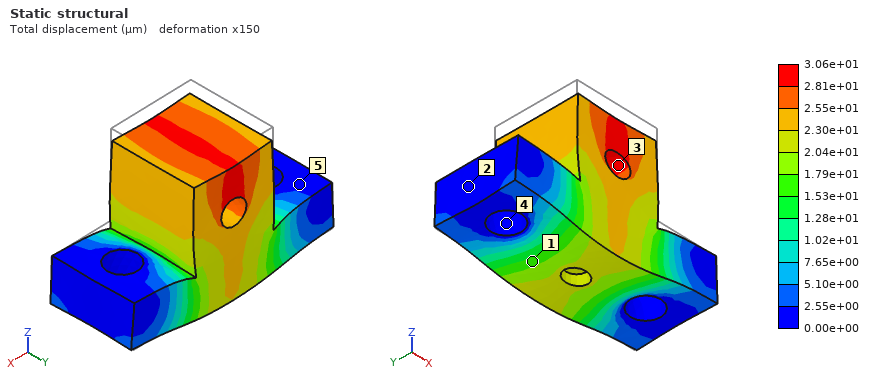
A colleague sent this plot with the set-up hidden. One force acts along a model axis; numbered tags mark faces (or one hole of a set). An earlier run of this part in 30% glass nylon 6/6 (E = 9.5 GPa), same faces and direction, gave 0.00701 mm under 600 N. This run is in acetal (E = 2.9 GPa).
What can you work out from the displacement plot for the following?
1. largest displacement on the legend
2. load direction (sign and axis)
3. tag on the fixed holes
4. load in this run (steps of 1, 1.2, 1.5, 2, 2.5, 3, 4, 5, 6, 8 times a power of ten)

3.06e+01 µm
-Z
4
800 N
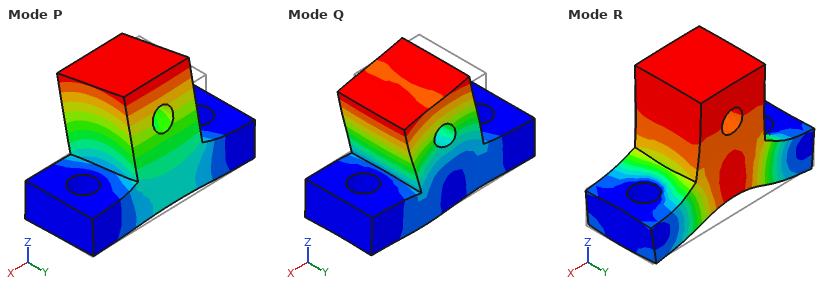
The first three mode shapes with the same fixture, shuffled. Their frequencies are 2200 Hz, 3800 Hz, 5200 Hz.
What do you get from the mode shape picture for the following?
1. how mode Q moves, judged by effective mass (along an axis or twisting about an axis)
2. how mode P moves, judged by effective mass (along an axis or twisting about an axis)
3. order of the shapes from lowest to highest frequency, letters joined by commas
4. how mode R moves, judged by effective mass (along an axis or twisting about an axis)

along X
along Y
P, Q, R
along Z
